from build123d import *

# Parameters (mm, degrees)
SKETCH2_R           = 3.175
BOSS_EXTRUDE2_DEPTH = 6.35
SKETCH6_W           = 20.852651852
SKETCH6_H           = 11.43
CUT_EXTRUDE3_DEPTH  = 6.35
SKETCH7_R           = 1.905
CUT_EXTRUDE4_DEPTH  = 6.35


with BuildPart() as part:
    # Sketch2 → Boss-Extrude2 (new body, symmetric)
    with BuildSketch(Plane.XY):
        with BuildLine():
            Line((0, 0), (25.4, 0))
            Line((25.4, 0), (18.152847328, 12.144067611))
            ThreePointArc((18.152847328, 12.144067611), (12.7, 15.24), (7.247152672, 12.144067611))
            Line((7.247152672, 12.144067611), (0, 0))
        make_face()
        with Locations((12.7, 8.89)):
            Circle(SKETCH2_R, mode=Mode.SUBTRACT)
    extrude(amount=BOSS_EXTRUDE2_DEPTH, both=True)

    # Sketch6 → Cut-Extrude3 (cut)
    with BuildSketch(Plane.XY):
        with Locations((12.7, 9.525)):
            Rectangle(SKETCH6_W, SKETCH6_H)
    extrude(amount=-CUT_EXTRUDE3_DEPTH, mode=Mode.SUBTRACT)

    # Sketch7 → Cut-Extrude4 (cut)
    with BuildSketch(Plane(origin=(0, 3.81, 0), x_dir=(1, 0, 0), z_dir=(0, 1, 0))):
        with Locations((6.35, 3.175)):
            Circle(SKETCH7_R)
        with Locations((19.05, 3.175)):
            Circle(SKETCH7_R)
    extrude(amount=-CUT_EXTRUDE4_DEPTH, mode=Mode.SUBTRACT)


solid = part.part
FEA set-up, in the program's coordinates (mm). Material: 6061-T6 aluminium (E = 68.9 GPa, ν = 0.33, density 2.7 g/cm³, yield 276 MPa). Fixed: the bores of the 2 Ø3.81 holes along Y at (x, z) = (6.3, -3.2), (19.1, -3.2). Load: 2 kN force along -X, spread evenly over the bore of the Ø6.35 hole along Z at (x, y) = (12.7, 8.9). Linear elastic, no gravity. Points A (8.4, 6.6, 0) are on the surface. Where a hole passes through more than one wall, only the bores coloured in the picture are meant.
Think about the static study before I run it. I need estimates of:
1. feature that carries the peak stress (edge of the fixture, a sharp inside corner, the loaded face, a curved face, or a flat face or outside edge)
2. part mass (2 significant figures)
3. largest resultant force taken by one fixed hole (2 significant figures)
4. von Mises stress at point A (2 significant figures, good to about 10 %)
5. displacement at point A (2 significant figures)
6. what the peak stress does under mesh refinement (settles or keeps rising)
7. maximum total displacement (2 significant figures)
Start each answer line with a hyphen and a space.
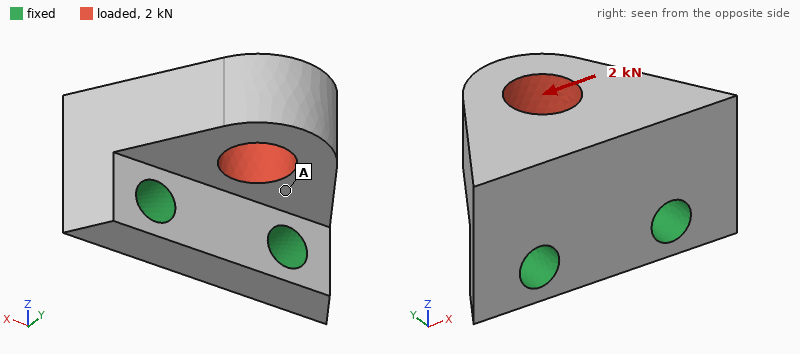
- edge of the fixture
- 4.9 g
- 1.5 kN
- 47 MPa
- 13 µm
- keeps rising
- 32 µm
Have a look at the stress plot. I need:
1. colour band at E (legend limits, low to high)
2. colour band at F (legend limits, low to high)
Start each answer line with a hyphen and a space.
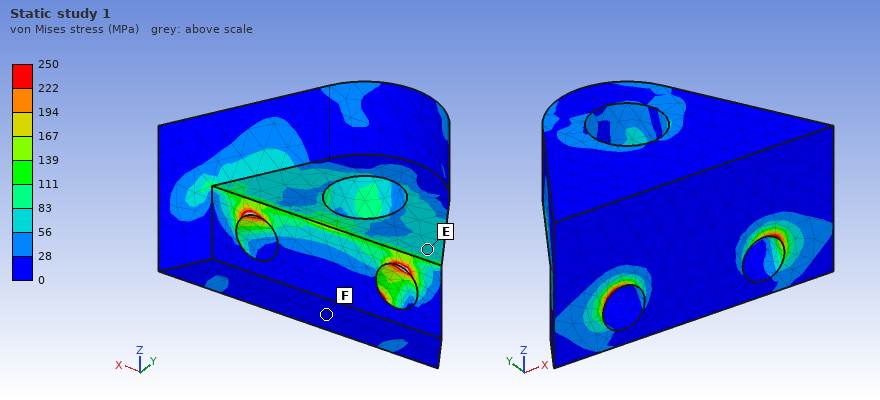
- 56 to 83 MPa
- 0 to 28 MPa
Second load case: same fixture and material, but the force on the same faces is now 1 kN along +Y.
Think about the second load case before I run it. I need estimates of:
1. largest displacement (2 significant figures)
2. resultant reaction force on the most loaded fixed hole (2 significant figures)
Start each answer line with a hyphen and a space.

- 36 µm
- 500 N
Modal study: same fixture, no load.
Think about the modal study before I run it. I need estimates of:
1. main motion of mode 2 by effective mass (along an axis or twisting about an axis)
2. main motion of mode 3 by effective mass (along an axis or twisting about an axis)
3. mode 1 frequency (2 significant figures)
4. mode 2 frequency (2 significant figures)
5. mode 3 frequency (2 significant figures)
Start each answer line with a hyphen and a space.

- along X
- along Y
- 15 kHz
- 29 kHz
- 44 kHz
